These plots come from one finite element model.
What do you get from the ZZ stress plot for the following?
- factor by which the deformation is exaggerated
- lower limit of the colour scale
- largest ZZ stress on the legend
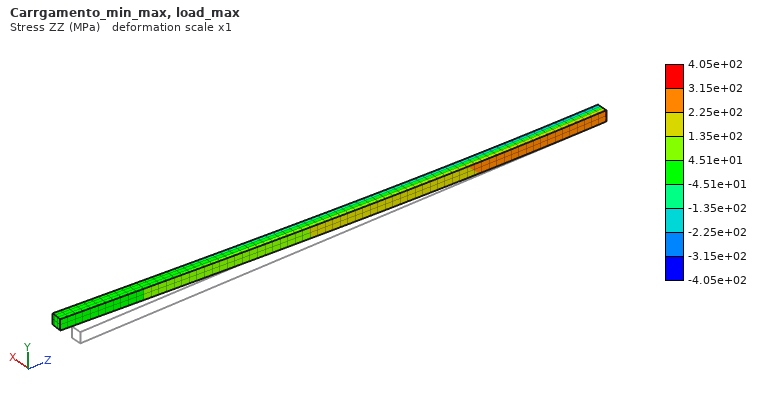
1
-4.05e+02 MPa
4.05e+02 MPa
